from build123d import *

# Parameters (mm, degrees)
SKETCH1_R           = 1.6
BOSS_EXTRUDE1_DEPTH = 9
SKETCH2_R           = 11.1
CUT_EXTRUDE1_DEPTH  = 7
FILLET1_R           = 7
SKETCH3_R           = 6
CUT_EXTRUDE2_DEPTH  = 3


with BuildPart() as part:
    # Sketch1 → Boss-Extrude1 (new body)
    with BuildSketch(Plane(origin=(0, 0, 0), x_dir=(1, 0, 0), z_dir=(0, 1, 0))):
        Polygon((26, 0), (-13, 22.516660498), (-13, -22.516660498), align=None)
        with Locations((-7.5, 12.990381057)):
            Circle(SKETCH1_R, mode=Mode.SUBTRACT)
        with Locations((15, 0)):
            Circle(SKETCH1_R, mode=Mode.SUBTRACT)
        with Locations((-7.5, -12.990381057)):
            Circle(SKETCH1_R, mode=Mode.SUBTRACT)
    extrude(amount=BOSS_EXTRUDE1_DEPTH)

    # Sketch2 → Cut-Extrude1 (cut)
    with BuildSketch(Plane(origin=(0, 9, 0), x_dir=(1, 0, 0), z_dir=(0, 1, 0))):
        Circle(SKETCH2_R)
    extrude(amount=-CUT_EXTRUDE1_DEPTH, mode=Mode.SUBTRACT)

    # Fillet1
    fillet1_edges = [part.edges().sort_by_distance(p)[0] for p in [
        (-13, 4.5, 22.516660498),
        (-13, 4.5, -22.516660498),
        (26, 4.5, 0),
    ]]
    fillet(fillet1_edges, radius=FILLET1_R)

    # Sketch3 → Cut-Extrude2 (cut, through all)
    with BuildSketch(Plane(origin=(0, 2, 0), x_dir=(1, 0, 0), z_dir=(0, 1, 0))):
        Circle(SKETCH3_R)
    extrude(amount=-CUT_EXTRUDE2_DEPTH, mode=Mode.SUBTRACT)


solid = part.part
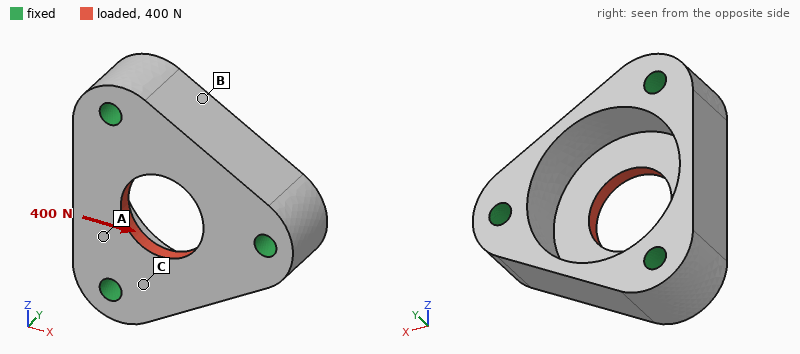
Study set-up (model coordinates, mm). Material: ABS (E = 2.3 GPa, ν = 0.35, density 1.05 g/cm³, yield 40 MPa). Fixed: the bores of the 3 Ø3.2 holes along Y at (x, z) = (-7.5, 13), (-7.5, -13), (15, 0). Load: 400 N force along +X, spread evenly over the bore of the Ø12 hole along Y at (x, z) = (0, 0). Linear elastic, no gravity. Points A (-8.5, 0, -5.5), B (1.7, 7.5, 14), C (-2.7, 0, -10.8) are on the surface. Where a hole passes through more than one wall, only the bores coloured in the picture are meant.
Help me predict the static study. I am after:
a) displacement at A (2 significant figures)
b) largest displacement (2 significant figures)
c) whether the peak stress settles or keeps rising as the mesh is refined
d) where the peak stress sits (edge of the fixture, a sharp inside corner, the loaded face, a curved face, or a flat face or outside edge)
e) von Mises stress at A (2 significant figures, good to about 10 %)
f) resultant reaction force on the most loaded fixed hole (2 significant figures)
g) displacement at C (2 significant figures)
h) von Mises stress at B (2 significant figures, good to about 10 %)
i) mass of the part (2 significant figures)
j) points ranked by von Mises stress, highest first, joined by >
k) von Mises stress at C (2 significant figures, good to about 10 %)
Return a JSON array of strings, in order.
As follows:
["37 µm", "66 µm", "keeps rising", "edge of the fixture", "6.4 MPa", "140 N", "13 µm", "1.3 MPa", "4.0 g", "A > C > B", "3.3 MPa"]
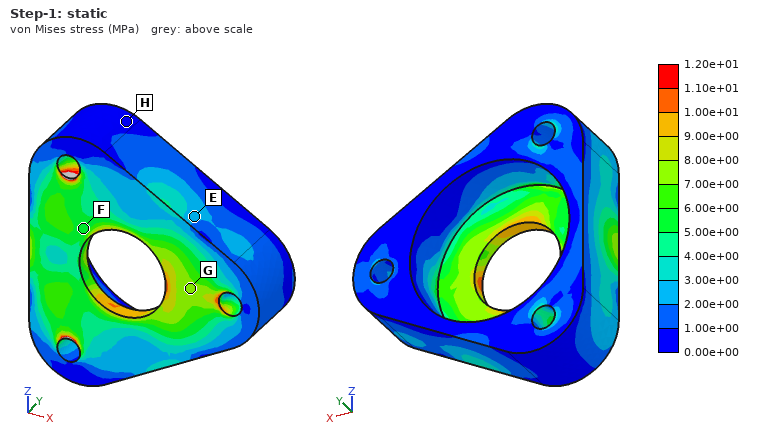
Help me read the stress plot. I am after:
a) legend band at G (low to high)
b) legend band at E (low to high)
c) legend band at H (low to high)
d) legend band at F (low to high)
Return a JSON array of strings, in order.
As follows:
["7.00e+00 to 8.00e+00 MPa", "2.00e+00 to 3.00e+00 MPa", "0.00e+00 to 1.00e+00 MPa", "5.00e+00 to 6.00e+00 MPa"]
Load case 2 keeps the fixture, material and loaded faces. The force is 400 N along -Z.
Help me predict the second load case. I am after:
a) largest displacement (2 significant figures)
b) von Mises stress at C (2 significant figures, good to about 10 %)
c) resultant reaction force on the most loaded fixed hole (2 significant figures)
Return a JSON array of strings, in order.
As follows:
["58 µm", "6.7 MPa", "140 N"]
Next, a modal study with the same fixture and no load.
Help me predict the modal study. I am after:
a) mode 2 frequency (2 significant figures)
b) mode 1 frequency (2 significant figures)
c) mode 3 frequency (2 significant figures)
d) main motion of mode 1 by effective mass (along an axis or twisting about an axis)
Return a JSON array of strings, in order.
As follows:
["14 kHz", "12 kHz", "14 kHz", "along Y"]
